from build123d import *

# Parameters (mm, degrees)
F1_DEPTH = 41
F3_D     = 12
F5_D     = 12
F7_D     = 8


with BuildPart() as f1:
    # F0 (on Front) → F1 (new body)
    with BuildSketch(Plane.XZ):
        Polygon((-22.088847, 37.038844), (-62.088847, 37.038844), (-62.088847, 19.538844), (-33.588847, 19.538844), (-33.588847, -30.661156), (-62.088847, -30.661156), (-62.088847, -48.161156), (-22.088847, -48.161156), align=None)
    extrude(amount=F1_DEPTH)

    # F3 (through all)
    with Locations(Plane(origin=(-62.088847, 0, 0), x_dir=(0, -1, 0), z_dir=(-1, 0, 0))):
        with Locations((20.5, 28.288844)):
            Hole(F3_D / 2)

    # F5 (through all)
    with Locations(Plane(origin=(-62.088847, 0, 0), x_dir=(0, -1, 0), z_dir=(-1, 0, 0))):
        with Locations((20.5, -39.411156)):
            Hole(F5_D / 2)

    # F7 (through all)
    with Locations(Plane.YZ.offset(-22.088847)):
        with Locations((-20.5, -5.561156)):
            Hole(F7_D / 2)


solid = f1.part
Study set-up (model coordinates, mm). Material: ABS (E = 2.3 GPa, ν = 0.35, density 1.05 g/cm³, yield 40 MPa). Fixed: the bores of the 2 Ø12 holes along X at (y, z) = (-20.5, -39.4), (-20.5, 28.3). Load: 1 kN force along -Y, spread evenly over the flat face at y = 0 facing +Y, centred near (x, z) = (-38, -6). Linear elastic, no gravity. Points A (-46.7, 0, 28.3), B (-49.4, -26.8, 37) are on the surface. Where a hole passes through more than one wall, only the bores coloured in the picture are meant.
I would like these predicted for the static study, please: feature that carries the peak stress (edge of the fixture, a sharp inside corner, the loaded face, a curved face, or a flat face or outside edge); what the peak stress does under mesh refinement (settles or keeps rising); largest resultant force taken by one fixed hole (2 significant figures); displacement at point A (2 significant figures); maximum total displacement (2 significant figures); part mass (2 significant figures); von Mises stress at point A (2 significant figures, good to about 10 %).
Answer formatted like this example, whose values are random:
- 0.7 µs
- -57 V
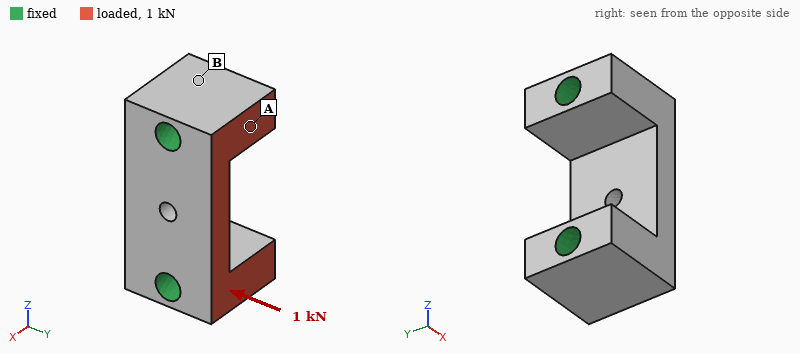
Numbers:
- edge of the fixture
- keeps rising
- 500 N
- 3.4 µm
- 14 µm
- 75 g
- 0.55 MPa
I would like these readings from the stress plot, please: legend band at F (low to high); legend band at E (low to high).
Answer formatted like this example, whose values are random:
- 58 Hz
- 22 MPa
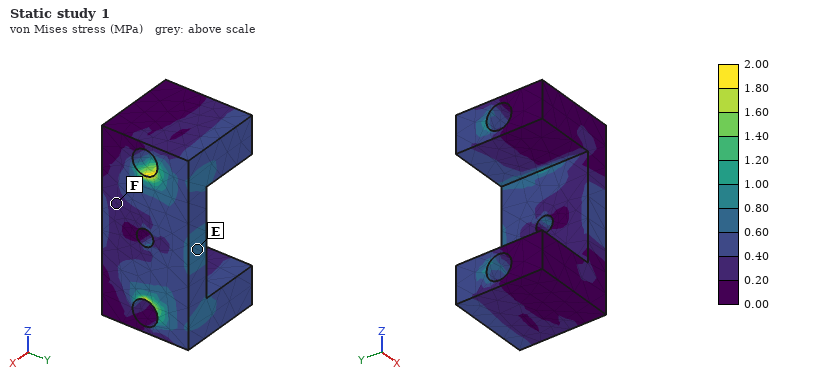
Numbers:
- 0.20 to 0.40 MPa
- 0.60 to 0.80 MPa
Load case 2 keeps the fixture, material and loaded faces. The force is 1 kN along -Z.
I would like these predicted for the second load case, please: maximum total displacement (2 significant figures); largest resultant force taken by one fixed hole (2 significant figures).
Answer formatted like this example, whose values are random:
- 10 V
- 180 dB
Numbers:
- 31 µm
- 520 N
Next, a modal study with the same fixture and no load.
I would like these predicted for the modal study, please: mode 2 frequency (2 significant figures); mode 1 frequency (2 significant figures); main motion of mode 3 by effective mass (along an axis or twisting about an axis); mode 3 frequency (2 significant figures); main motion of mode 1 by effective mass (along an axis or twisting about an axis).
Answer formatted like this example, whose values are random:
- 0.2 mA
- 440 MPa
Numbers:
- 4900 Hz
- 4200 Hz
- along Y
- 5700 Hz
- along X
